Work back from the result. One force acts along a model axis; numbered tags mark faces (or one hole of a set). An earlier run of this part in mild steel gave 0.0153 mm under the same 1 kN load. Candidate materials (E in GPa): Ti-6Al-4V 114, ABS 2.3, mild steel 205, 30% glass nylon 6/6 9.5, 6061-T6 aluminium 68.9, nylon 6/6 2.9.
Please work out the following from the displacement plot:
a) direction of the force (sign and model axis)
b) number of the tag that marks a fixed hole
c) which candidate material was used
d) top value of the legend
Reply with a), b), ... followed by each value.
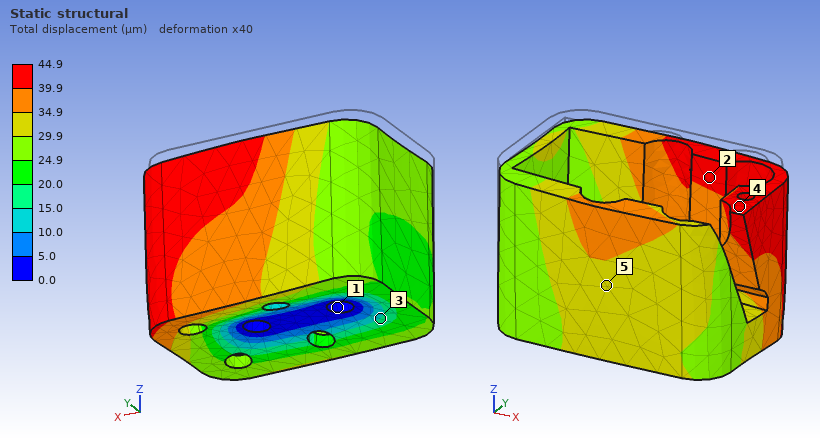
a) -Z
b) 1
c) 6061-T6 aluminium
d) 44.9 µm
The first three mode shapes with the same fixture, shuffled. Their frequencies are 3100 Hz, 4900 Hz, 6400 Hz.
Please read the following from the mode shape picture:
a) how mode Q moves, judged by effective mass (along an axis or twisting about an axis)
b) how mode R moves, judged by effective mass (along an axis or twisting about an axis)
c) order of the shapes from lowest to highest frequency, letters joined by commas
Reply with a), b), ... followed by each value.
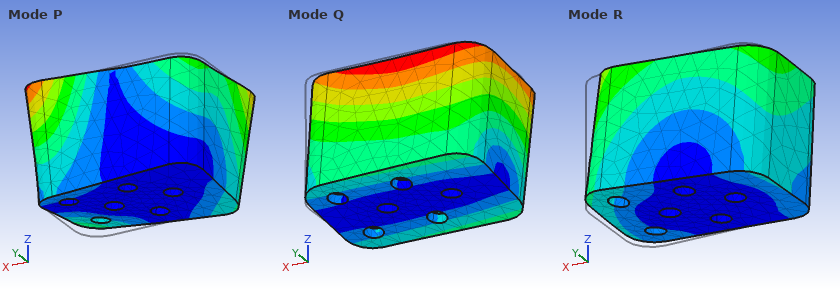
a) along Y
b) along X
c) Q, R, P
